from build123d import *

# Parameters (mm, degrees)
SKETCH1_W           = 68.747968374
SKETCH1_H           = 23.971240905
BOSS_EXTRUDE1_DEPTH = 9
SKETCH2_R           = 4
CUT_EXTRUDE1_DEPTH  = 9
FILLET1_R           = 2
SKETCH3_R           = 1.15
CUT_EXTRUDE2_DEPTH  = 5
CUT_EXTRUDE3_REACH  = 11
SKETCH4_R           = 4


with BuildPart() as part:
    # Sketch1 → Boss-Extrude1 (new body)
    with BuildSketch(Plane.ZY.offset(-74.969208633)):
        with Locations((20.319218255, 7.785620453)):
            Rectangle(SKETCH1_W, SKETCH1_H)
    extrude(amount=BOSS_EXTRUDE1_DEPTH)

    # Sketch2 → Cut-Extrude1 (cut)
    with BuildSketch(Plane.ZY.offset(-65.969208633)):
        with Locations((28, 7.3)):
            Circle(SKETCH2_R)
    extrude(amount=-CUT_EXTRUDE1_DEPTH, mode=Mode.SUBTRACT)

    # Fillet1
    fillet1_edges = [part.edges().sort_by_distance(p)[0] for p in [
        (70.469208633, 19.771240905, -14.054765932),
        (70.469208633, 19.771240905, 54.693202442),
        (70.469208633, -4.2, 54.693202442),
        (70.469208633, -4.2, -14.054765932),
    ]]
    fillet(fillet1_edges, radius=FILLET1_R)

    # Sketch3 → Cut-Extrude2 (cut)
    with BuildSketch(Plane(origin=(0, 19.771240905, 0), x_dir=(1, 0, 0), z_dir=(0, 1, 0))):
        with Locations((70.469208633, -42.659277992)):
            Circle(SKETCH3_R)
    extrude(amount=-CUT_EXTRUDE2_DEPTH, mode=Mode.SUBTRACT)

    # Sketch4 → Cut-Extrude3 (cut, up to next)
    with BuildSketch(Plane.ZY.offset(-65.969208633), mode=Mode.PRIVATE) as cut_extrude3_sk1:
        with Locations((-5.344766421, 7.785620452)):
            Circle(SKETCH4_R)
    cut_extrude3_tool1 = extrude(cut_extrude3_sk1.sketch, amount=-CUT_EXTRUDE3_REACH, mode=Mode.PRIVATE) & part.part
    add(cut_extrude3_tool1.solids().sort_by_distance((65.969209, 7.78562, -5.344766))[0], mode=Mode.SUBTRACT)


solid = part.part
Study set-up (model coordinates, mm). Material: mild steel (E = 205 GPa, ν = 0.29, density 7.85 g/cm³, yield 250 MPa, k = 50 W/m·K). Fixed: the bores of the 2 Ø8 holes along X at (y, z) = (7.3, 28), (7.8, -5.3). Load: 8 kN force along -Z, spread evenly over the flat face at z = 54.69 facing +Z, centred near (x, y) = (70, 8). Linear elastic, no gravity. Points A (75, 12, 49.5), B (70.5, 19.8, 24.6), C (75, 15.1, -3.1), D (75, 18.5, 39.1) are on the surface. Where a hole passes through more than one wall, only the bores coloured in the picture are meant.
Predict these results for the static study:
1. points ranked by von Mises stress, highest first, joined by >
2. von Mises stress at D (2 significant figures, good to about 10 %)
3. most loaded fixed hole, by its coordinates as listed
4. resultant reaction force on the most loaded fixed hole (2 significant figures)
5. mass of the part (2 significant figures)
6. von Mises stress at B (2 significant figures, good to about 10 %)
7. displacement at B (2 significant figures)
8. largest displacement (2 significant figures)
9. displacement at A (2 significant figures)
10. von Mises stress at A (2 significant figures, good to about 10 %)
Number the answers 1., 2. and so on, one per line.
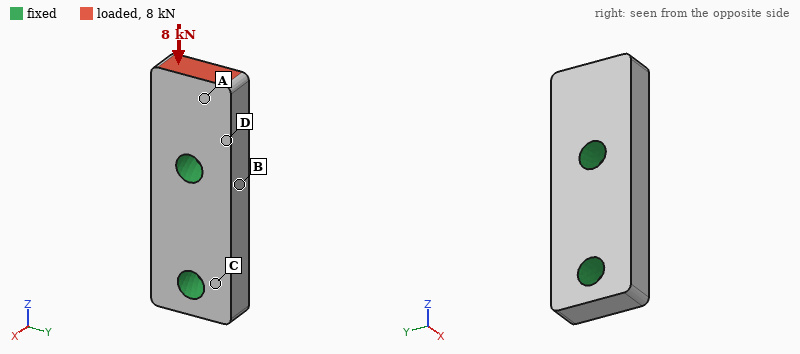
1. A > D > B > C
2. 31 MPa
3. (7.3, 28)
4. 7.4 kN
5. 110 g
6. 19 MPa
7. 1.00 µm
8. 5.6 µm
9. 4.5 µm
10. 46 MPa
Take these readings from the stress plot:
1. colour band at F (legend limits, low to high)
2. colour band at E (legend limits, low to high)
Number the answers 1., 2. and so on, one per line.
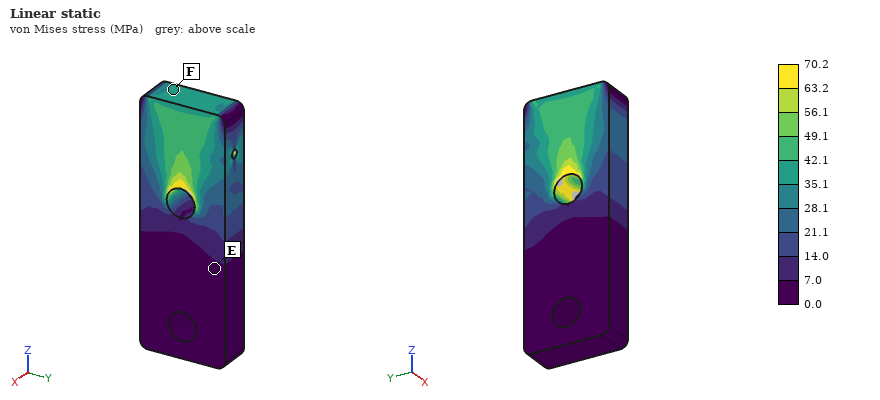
1. 35.1 to 42.1 MPa
2. 0.0 to 7.0 MPa
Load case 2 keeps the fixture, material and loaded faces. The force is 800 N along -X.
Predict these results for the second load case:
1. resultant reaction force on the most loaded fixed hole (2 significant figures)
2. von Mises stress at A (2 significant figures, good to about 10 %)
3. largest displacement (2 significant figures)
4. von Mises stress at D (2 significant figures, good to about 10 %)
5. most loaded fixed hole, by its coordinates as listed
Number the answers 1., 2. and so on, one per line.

1. 870 N
2. 15 MPa
3. 16 µm
4. 36 MPa
5. (7.3, 28)
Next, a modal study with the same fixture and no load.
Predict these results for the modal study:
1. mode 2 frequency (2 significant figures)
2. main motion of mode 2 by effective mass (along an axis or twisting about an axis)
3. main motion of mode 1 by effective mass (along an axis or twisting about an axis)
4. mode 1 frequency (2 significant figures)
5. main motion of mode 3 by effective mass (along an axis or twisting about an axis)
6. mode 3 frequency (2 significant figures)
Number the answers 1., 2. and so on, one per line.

1. 16 kHz
2. along Y
3. along X
4. 11 kHz
5. twisting about Z
6. 20 kHz
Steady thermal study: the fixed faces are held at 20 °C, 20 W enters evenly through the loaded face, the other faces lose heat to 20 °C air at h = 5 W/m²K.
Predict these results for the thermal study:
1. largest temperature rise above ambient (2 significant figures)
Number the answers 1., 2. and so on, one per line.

1. 49 K
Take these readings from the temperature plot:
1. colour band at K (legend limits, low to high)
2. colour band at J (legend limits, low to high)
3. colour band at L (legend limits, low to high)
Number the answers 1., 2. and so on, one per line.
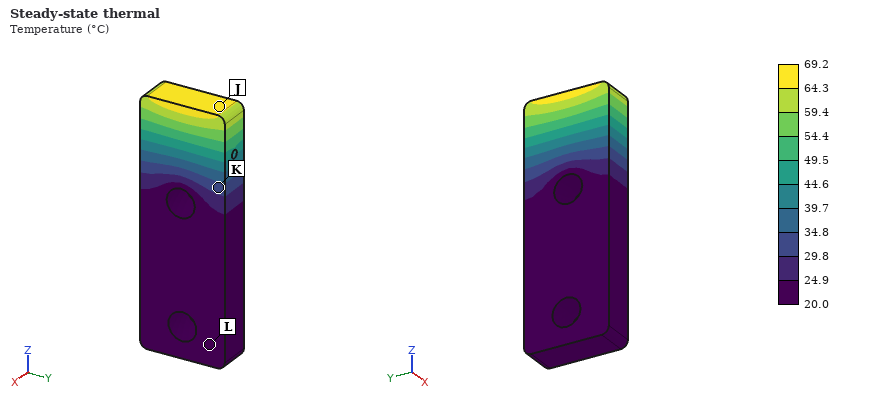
1. 29.8 to 34.8 °C
2. 64.3 to 69.2 °C
3. 20.0 to 24.9 °C
